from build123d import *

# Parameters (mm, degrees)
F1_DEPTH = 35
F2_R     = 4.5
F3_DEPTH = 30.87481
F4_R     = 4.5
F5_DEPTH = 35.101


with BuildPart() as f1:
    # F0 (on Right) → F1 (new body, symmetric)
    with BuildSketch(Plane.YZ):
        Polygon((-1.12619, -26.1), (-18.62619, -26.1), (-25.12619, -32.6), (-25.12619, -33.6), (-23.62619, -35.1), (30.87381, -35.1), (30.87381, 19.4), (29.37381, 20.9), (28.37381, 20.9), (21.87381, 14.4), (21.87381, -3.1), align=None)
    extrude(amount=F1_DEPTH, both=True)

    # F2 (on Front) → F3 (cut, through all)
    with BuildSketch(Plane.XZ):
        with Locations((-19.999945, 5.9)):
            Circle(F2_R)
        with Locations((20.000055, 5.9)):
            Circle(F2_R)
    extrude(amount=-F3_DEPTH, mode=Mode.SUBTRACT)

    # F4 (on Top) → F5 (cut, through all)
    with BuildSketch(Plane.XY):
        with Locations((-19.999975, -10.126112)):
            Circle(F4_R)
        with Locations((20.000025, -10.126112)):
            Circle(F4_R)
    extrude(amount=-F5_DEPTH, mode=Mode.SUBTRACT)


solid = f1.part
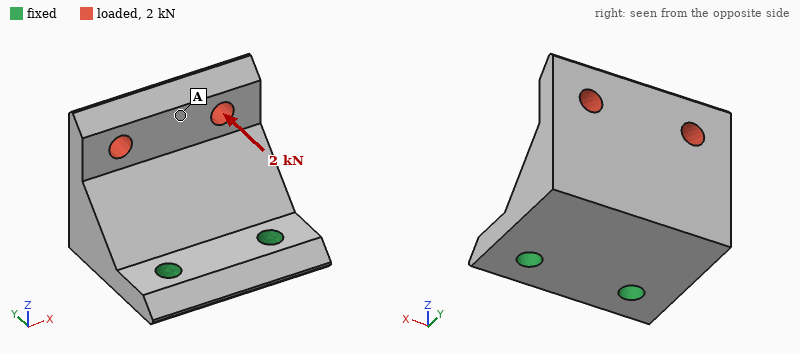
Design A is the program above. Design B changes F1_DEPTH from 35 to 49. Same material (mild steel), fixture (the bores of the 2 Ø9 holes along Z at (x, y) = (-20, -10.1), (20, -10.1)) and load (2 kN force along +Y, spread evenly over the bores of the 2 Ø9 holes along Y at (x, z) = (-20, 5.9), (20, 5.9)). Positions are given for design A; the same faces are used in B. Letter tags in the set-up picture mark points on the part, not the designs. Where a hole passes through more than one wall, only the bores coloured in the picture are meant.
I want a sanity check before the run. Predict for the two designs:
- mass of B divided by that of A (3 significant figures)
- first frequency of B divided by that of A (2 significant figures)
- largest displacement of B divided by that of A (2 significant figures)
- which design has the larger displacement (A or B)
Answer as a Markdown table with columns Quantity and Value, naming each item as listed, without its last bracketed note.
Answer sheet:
| Quantity | Value |
|---|---|
| mass of B divided by that of A | 1.41 |
| first frequency of B divided by that of A | 0.91 |
| largest displacement of B divided by that of A | 0.83 |
| which design has the larger displacement | A |
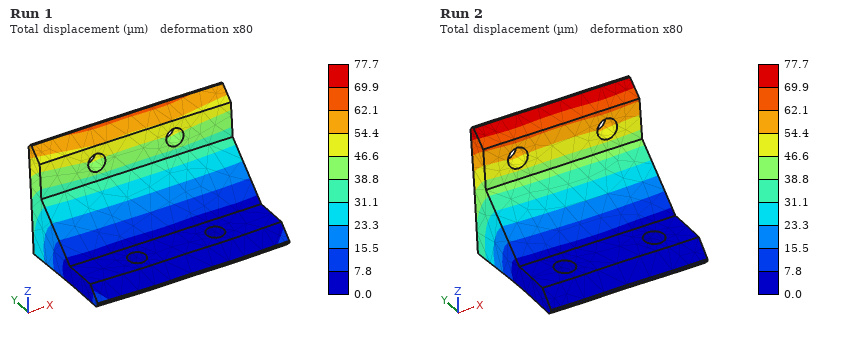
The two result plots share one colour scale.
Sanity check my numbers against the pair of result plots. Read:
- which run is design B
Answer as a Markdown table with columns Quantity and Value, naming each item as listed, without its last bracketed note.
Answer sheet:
| Quantity | Value |
|---|---|
| which run is design B | Run 1 |
